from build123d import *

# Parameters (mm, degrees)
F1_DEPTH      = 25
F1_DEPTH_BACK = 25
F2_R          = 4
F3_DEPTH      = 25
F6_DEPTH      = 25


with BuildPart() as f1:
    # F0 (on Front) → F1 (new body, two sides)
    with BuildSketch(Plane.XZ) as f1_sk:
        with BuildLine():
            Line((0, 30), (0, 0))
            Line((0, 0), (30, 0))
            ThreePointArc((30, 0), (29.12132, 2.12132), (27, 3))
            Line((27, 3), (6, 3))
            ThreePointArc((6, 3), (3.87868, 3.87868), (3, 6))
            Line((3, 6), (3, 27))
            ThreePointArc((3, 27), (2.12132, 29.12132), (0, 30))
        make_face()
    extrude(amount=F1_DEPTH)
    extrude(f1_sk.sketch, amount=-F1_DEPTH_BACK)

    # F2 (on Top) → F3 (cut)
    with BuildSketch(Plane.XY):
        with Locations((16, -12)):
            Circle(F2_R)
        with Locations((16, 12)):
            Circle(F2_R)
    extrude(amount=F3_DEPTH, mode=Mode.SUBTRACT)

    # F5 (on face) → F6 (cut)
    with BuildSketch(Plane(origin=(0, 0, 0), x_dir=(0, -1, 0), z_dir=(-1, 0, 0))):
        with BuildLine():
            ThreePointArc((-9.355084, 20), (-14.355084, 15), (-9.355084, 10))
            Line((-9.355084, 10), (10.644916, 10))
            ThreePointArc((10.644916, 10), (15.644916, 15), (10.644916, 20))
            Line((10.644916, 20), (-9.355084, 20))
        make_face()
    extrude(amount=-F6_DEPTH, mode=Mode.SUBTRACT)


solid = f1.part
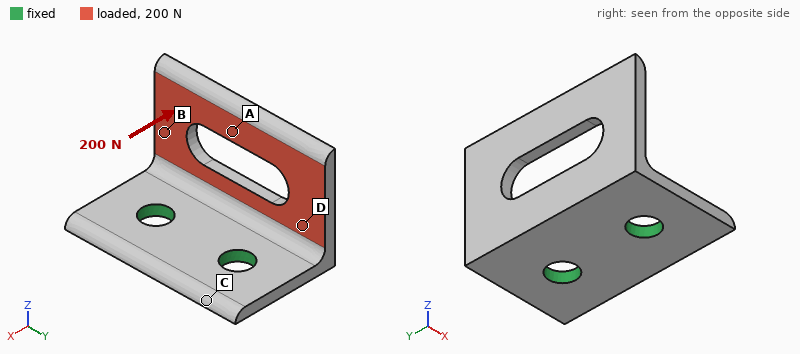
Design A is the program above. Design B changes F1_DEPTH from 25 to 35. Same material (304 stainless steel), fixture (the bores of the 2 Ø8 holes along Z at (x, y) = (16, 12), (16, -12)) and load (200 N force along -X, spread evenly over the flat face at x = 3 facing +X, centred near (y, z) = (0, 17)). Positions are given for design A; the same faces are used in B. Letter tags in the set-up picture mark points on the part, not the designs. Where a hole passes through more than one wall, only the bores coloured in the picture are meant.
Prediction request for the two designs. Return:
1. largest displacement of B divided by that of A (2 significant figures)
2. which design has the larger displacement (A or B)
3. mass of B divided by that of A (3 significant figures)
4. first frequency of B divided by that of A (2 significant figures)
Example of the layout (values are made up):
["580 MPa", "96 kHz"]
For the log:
["0.81", "A", "1.23", "0.99"]
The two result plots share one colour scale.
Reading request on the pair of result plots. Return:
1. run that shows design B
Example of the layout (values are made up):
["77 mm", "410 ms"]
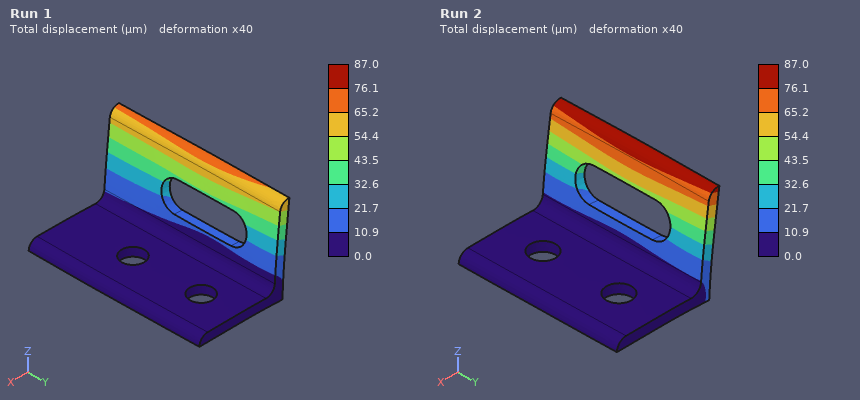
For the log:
["Run 1"]
